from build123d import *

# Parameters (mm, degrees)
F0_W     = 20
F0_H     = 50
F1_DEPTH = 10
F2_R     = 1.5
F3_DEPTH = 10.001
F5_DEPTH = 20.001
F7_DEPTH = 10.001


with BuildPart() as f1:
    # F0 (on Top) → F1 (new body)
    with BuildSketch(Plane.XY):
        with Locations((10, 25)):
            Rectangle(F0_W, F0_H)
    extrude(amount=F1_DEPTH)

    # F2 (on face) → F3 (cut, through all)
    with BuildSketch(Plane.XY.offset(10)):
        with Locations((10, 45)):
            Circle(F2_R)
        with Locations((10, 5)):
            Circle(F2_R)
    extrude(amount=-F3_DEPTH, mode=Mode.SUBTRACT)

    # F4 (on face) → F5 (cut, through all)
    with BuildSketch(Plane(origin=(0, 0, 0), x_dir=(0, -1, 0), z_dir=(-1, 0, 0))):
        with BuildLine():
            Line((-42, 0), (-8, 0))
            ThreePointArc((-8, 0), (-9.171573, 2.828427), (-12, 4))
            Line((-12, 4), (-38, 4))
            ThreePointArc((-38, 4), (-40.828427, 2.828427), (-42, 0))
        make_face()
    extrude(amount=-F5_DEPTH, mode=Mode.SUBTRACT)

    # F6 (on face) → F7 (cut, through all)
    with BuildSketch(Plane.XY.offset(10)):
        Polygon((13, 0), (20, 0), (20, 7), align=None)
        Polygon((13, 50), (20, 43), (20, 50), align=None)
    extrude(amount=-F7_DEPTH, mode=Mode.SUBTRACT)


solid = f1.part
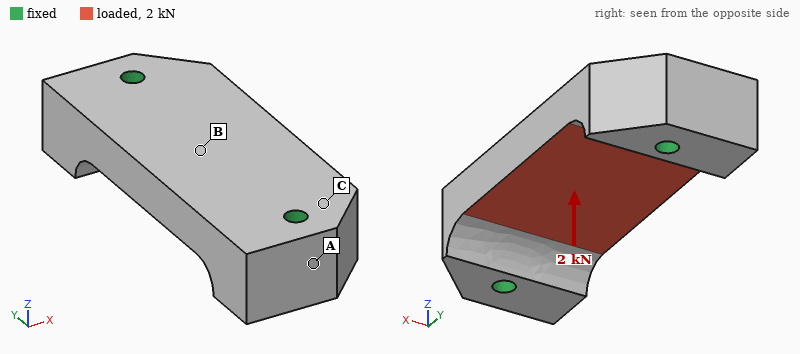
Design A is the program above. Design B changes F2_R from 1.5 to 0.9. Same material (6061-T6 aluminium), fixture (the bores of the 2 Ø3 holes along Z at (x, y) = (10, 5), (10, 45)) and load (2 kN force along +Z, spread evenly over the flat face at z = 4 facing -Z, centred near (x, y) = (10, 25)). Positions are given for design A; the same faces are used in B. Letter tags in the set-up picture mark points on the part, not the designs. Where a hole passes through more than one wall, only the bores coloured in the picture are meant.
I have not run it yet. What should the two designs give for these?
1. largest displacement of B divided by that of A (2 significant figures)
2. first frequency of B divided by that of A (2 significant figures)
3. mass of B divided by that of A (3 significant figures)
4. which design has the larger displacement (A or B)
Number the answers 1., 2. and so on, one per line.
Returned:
1. 1.1
2. 0.93
3. 1.01
4. B
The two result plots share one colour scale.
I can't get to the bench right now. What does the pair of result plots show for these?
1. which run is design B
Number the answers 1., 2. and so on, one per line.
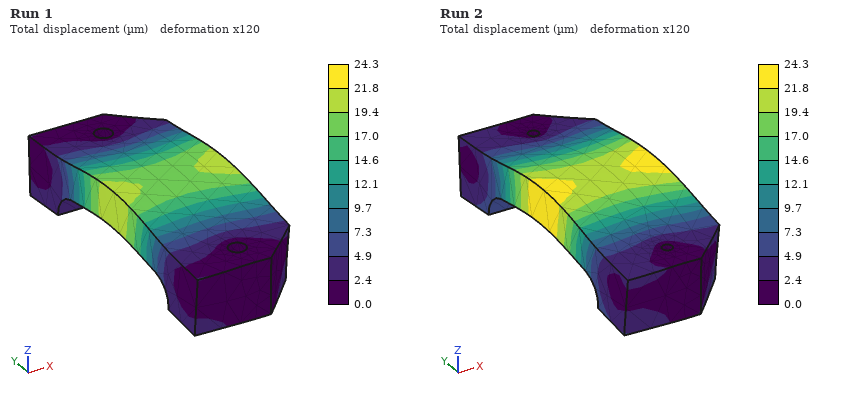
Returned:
1. Run 2
